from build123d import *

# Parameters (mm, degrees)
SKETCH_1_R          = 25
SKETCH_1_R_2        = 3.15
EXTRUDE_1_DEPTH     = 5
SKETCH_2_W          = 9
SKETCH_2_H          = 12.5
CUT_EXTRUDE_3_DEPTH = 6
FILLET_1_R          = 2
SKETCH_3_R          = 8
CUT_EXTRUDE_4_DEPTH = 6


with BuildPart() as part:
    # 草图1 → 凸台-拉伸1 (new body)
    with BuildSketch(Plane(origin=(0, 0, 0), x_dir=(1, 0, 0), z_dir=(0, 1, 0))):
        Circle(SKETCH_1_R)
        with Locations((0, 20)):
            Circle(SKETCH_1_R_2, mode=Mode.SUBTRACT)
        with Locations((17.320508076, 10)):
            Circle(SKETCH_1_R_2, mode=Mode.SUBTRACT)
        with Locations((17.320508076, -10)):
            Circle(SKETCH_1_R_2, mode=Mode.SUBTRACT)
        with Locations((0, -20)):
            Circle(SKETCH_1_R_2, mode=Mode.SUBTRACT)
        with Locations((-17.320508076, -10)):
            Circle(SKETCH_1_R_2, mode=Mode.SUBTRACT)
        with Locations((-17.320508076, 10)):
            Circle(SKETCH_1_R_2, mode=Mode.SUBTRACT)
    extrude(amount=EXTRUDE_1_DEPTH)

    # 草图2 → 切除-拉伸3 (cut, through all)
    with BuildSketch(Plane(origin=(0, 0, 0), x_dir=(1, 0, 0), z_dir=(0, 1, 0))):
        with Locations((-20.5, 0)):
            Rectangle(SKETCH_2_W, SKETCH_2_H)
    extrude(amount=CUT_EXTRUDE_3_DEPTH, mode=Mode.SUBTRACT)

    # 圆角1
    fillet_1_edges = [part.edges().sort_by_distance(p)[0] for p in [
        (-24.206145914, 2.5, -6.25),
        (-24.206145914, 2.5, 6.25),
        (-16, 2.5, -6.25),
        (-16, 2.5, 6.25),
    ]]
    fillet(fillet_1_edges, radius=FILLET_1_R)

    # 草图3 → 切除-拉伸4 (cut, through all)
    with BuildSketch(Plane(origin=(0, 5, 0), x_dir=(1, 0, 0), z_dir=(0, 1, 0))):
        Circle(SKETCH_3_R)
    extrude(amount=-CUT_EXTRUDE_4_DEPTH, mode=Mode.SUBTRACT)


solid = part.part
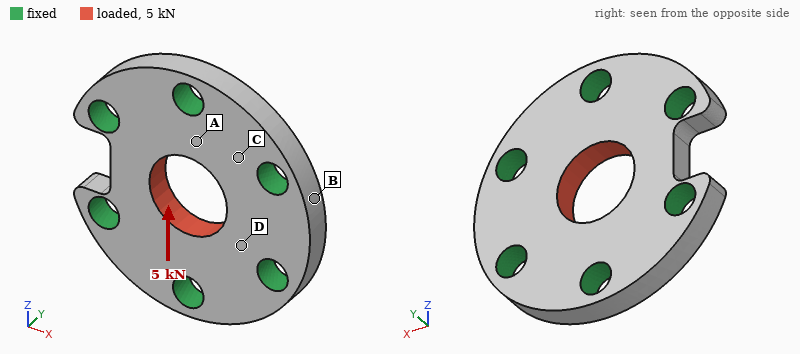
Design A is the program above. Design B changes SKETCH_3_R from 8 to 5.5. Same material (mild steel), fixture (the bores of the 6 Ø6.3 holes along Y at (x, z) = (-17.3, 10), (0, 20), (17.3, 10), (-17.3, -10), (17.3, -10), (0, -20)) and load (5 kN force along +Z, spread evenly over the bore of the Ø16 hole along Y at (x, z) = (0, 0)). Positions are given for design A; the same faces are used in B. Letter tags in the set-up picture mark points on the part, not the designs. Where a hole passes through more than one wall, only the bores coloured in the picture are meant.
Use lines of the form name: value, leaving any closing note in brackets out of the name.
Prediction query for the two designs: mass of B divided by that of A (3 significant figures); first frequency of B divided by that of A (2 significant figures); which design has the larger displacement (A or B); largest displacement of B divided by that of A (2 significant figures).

mass of B divided by that of A: 1.07
first frequency of B divided by that of A: 0.82
which design has the larger displacement: B
largest displacement of B divided by that of A: 1.4
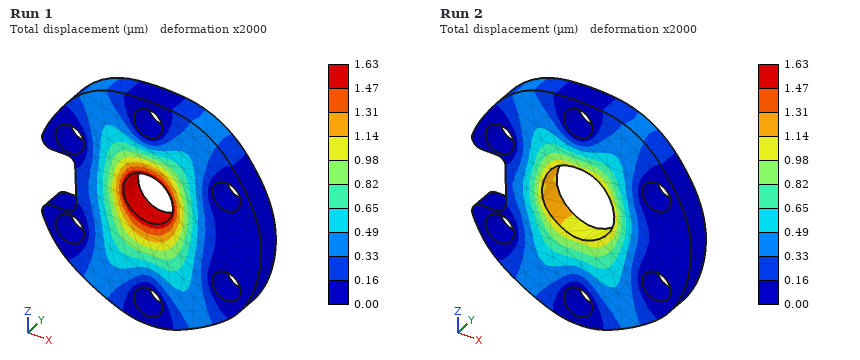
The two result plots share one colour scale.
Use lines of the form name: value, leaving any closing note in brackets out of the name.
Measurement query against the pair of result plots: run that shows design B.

run that shows design B: Run 1
